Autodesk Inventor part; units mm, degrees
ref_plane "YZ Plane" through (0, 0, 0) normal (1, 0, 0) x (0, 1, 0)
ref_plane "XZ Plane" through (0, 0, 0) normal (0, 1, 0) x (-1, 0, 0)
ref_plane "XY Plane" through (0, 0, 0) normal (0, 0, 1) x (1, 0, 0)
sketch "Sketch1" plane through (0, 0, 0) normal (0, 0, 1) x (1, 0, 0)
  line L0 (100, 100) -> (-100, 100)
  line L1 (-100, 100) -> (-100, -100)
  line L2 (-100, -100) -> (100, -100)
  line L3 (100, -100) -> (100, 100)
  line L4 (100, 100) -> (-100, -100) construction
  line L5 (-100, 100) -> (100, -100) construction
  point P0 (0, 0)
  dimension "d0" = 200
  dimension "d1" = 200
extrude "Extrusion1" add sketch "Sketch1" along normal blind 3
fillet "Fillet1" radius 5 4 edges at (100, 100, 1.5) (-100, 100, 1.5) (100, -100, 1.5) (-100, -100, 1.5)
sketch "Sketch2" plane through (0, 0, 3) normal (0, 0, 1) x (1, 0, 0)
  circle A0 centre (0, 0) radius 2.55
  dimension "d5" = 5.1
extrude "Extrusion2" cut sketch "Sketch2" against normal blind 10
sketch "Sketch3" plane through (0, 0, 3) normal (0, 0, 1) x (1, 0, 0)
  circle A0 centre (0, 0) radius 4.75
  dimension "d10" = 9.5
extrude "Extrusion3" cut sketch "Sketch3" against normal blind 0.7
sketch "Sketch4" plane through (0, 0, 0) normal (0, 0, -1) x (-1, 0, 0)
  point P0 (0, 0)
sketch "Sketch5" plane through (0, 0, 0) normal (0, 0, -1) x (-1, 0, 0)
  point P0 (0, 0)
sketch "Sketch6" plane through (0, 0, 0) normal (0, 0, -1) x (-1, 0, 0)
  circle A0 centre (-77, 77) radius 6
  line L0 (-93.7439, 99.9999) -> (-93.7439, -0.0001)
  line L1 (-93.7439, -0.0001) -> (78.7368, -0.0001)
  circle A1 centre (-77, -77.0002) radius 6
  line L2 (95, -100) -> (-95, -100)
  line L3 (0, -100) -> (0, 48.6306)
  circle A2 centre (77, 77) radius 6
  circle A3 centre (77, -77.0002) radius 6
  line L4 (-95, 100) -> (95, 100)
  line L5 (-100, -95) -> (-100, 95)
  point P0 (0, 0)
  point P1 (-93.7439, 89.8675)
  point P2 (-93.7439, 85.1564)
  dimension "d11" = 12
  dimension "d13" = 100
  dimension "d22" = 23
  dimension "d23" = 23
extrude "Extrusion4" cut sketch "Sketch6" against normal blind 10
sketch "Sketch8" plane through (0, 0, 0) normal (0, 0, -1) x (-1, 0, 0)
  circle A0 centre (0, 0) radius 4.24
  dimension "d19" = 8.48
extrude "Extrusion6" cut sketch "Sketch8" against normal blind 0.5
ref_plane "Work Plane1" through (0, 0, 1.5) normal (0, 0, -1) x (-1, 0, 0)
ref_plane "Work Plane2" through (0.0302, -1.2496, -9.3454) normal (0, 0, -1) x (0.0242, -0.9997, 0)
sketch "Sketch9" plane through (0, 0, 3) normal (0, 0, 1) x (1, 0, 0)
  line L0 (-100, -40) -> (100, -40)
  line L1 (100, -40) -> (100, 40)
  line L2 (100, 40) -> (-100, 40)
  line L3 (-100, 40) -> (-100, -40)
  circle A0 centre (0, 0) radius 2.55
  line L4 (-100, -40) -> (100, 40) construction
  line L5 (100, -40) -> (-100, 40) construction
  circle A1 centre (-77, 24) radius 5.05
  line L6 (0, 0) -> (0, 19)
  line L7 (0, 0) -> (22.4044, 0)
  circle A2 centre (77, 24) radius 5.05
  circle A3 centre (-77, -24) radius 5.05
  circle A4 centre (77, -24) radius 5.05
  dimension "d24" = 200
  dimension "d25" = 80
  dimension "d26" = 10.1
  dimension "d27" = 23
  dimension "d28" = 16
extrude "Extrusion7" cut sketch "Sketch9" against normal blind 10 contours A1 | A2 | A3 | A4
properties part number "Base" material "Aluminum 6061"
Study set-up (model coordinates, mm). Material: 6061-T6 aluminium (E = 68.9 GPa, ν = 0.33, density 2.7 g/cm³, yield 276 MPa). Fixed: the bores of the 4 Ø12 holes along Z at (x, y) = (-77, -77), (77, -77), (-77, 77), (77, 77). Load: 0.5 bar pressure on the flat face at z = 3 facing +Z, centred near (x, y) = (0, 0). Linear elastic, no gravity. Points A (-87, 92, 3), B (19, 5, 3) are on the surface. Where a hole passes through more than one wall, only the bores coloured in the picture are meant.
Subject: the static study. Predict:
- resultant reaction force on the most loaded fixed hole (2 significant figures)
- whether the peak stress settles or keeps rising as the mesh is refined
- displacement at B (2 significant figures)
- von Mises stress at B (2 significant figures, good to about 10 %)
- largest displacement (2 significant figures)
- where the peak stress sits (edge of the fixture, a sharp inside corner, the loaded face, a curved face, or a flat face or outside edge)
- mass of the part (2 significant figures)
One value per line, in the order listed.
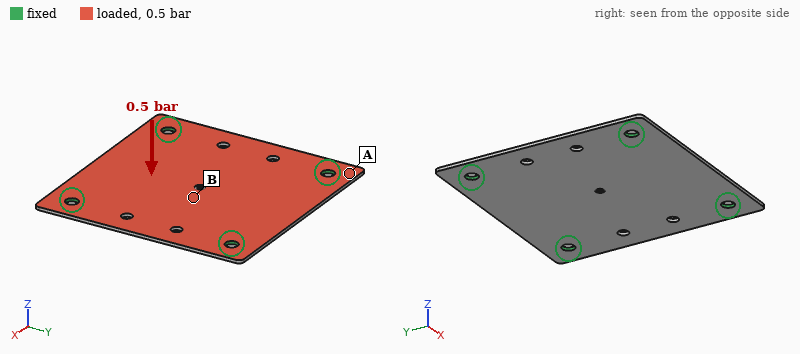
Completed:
490 N
keeps rising
0.95 mm
36 MPa
1.0 mm
edge of the fixture
320 g
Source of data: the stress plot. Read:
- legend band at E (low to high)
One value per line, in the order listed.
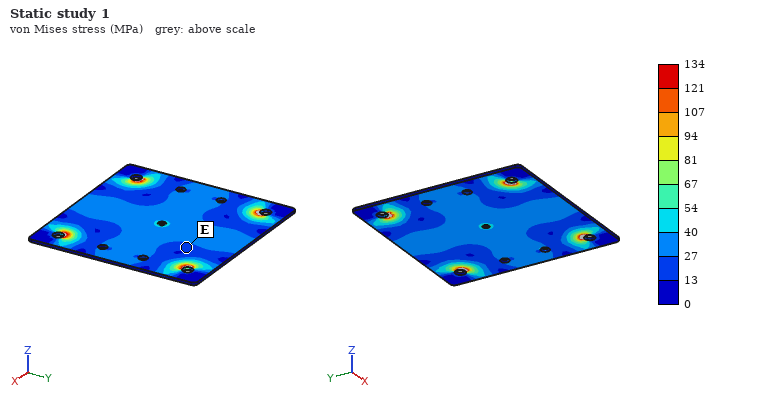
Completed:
13 to 27 MPa
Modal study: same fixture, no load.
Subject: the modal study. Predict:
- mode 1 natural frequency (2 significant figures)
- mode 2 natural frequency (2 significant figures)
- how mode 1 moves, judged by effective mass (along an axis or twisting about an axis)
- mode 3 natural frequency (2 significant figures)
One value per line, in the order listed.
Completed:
490 Hz
780 Hz
along Z
780 Hz
